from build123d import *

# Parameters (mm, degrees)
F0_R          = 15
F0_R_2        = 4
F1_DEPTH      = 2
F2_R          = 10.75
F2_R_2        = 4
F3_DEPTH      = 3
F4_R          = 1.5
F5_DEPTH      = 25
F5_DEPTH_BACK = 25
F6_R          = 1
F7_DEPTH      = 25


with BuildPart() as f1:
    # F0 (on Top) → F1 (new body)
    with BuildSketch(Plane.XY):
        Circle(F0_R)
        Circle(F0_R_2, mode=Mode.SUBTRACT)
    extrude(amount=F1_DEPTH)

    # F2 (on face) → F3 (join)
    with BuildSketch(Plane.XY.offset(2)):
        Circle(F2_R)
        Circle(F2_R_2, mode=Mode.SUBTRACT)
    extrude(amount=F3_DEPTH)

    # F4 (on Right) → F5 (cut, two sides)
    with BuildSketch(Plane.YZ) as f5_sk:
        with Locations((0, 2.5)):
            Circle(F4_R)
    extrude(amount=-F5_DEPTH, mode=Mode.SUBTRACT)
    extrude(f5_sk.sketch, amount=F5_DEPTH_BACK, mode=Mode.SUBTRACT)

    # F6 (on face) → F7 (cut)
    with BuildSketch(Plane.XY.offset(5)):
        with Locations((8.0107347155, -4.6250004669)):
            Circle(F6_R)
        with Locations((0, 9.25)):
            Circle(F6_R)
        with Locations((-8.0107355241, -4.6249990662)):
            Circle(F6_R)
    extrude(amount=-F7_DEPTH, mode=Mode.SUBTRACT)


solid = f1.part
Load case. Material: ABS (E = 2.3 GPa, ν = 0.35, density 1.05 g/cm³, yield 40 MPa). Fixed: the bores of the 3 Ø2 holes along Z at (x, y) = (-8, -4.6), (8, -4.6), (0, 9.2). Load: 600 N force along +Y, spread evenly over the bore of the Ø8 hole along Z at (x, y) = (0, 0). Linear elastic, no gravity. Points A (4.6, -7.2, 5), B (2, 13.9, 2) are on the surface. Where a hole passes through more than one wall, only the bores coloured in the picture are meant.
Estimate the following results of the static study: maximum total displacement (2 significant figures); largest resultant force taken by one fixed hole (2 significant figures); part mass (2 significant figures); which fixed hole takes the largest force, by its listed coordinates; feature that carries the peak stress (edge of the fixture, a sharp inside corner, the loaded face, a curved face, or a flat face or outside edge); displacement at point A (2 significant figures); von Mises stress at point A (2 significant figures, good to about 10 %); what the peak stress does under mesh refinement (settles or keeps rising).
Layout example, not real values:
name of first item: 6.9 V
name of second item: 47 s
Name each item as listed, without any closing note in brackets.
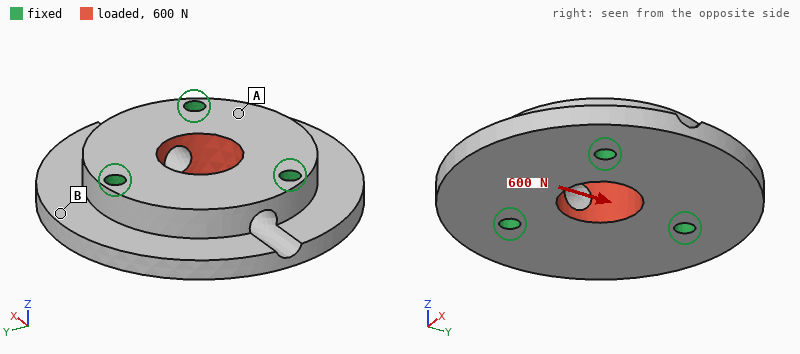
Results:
maximum total displacement: 40 µm
largest resultant force taken by one fixed hole: 220 N
part mass: 2.2 g
which fixed hole takes the largest force, by its listed coordinates: (0, 9.2)
feature that carries the peak stress: edge of the fixture
displacement at point A: 21 µm
von Mises stress at point A: 5.4 MPa
what the peak stress does under mesh refinement: keeps rising
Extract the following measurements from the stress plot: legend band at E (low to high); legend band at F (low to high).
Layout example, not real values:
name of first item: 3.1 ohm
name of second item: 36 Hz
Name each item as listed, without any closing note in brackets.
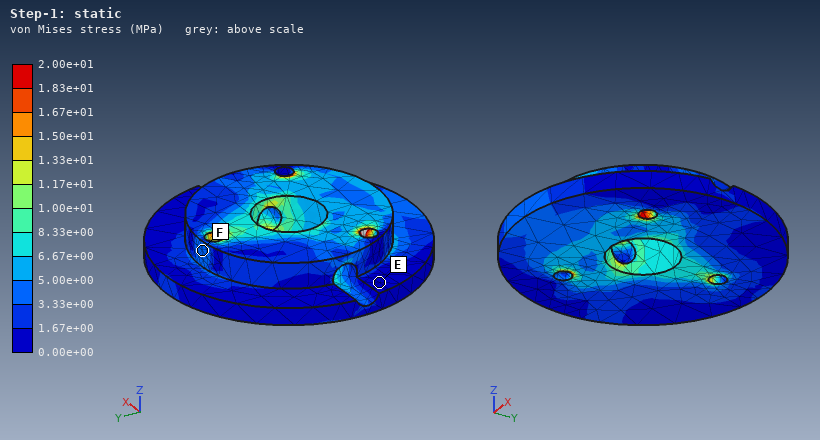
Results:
legend band at E: 0.00e+00 to 1.67e+00 MPa
legend band at F: 3.33e+00 to 5.00e+00 MPa
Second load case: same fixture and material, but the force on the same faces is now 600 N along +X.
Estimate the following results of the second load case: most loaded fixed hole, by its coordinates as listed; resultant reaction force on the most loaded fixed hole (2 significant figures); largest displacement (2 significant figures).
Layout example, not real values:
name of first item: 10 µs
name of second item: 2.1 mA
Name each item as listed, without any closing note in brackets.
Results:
most loaded fixed hole, by its coordinates as listed: (0, 9.2)
resultant reaction force on the most loaded fixed hole: 220 N
largest displacement: 36 µm
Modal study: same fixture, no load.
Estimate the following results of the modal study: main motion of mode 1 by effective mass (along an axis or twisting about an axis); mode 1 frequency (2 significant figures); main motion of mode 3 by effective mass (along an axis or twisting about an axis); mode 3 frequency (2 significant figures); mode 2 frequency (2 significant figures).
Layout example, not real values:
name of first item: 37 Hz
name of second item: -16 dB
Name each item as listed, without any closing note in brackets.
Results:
main motion of mode 1 by effective mass: twisting about Y
mode 1 frequency: 8600 Hz
main motion of mode 3 by effective mass: along Z
mode 3 frequency: 10 kHz
mode 2 frequency: 9100 Hz
